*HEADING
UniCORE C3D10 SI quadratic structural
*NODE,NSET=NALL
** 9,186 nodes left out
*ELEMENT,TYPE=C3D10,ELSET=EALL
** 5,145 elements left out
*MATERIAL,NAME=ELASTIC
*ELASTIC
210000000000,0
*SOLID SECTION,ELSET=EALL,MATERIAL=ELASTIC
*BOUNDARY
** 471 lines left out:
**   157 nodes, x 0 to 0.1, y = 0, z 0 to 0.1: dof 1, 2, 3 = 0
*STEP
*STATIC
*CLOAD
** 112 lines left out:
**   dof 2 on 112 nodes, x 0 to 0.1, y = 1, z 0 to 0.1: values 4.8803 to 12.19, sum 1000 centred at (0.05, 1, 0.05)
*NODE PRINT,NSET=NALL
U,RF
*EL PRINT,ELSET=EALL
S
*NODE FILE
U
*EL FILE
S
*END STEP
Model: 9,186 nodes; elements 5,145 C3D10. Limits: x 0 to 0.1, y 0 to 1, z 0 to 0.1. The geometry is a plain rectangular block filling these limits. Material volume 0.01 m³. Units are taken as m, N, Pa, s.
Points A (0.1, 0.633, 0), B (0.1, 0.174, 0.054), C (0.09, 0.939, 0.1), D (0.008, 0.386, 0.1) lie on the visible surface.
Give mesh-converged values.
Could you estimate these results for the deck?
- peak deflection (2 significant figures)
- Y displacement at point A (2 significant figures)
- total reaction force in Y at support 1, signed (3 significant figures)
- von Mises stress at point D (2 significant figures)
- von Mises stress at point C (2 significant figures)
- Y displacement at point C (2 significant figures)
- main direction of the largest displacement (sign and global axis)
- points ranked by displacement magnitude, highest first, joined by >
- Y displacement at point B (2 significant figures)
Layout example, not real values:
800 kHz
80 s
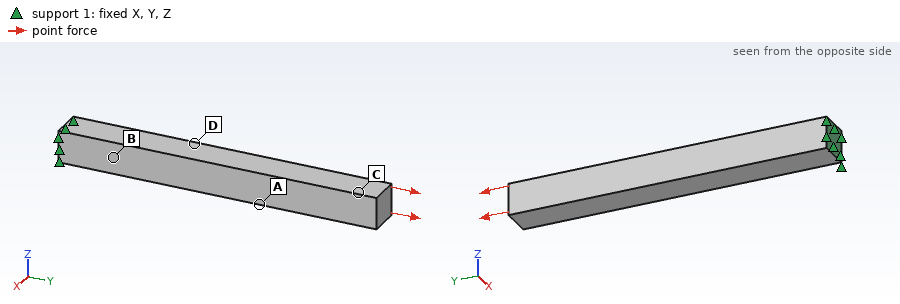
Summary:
4.9e-07 m
3.0e-07 m
-1000 N
100000 Pa
1.0e+05 Pa
4.5e-07 m
+Y
C > A > D > B
8.3e-08 m
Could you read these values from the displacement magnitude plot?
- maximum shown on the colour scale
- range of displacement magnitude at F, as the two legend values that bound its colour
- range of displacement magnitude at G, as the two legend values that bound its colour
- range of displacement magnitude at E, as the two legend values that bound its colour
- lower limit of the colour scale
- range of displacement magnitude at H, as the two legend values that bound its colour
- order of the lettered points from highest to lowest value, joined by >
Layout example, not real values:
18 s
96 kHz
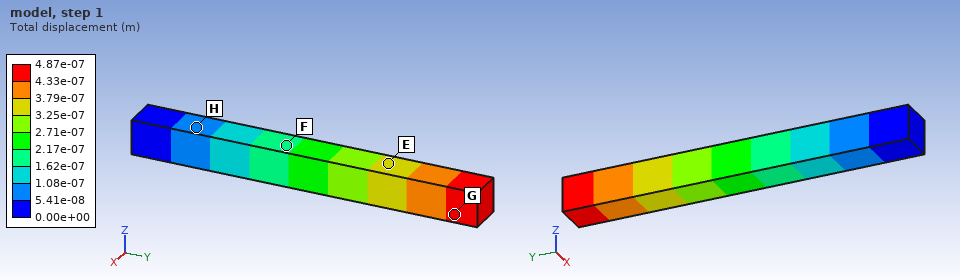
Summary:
4.87e-07 m
1.62e-07 to 2.17e-07 m
4.33e-07 to 4.87e-07 m
3.25e-07 to 3.79e-07 m
0.00e+00 m
5.41e-08 to 1.08e-07 m
G > E > F > H
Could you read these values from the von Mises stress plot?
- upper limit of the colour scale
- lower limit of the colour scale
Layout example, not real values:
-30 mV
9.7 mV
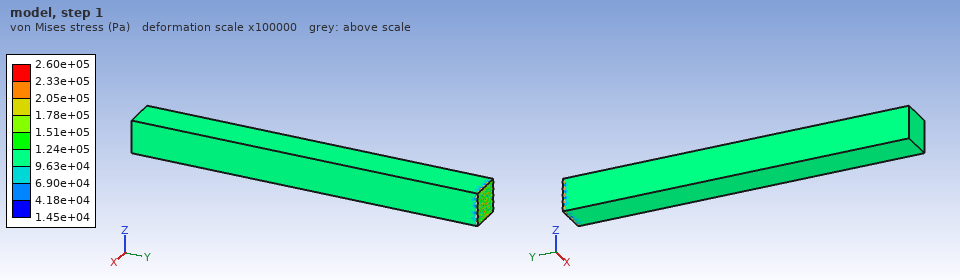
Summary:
2.60e+05 Pa
1.45e+04 Pa
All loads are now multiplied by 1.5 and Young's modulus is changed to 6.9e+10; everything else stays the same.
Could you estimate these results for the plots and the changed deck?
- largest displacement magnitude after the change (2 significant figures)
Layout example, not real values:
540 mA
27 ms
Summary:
2.2e-06 m
